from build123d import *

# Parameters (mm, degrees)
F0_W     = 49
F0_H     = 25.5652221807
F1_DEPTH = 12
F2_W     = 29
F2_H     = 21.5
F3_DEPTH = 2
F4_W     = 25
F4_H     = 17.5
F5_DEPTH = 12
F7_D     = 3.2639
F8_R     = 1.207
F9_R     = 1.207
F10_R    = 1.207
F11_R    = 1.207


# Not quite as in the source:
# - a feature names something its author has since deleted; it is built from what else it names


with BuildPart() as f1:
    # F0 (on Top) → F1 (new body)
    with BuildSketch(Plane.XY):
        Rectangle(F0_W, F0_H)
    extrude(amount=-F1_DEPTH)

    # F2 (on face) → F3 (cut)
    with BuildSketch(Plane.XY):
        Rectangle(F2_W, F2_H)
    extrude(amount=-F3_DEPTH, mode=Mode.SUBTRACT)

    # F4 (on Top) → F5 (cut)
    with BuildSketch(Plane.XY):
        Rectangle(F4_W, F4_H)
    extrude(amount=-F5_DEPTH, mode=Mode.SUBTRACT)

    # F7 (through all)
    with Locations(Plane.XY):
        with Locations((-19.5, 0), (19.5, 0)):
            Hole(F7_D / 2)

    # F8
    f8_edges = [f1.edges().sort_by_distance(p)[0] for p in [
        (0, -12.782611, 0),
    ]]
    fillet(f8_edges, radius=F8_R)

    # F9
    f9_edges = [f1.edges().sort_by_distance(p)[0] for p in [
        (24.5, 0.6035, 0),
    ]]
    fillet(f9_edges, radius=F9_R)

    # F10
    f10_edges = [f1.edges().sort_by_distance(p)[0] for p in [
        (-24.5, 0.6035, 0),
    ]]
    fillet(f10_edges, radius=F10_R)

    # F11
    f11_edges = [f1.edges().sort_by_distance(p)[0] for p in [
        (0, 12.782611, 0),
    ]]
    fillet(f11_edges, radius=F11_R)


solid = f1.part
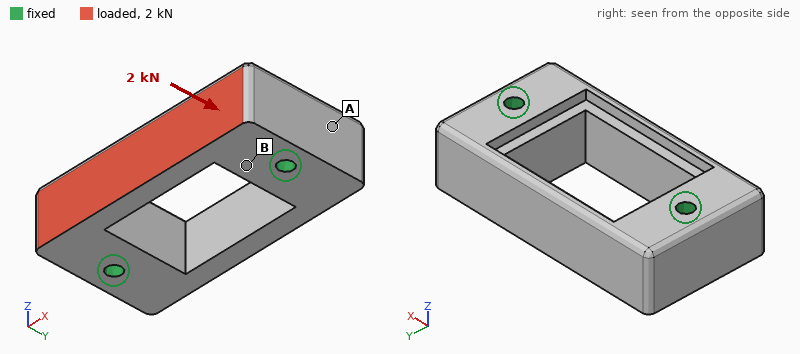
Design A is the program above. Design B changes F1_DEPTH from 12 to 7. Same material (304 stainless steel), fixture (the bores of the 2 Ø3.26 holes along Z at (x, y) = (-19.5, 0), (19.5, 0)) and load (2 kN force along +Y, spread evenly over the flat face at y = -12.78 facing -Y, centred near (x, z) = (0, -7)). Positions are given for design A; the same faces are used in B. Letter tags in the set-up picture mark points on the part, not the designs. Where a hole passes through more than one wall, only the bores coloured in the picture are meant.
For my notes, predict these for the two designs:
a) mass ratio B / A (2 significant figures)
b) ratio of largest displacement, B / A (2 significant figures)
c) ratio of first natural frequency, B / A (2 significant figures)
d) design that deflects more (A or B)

0.56
1.9
0.88
B
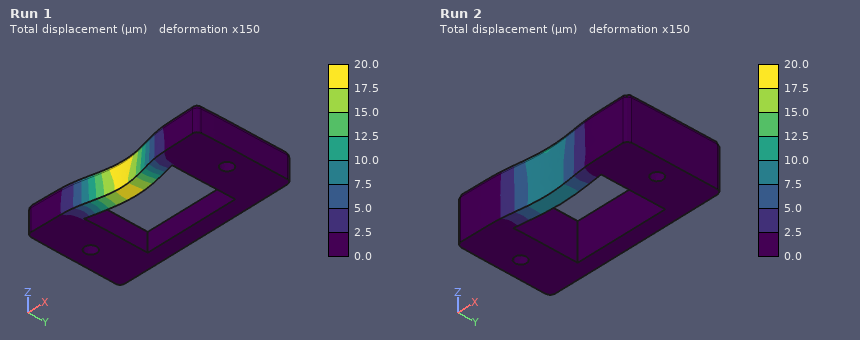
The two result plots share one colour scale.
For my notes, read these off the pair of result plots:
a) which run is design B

Run 1
